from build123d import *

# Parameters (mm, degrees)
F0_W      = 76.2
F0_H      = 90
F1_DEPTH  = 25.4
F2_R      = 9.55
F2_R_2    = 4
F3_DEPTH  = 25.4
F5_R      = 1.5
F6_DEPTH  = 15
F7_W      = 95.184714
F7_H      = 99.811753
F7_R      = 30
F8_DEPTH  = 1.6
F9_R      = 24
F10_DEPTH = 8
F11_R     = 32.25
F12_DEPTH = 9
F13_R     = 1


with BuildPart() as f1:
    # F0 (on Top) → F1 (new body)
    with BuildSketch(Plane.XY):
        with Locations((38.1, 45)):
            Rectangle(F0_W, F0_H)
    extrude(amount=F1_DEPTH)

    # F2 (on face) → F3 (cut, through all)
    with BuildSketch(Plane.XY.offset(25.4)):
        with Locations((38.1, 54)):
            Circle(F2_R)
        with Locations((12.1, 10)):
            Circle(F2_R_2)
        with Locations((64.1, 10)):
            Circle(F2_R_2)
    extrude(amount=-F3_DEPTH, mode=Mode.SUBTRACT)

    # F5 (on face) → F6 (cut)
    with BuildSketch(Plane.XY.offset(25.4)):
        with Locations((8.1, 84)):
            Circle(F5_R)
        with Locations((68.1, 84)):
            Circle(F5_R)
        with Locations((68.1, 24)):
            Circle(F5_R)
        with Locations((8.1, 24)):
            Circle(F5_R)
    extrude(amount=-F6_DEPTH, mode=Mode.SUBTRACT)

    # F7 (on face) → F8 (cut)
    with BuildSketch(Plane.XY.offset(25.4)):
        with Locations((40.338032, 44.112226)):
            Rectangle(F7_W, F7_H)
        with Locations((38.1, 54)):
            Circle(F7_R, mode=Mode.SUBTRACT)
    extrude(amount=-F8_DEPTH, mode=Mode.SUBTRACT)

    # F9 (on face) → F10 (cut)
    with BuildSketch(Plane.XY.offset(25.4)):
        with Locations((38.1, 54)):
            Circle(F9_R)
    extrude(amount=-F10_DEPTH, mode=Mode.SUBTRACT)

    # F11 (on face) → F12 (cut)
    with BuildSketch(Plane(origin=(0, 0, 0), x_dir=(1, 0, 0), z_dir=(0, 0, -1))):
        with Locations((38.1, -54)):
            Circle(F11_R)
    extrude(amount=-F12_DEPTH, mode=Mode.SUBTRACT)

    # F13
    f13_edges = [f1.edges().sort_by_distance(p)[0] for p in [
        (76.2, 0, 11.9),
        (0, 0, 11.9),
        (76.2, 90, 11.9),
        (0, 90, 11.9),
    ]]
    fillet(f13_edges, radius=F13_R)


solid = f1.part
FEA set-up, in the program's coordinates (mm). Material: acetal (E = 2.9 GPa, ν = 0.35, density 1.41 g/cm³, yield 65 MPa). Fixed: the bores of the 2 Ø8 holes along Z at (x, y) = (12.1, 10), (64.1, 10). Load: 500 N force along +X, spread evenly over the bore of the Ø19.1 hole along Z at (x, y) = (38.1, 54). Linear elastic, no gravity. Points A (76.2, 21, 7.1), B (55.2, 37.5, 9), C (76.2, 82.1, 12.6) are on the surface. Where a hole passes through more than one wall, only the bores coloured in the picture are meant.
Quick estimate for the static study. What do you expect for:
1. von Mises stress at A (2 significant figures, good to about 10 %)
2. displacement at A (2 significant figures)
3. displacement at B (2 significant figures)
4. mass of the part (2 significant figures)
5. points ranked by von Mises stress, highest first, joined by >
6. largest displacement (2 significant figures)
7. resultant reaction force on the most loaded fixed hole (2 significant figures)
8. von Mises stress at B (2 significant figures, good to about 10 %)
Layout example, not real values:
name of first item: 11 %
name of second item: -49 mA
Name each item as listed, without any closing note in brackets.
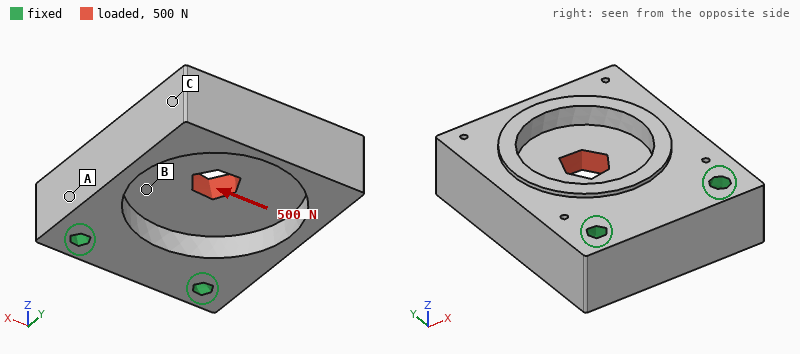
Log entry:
von Mises stress at A: 0.87 MPa
displacement at A: 9.3 µm
displacement at B: 18 µm
mass of the part: 170 g
points ranked by von Mises stress, highest first, joined by >: B > A > C
largest displacement: 59 µm
resultant reaction force on the most loaded fixed hole: 450 N
von Mises stress at B: 1.3 MPa
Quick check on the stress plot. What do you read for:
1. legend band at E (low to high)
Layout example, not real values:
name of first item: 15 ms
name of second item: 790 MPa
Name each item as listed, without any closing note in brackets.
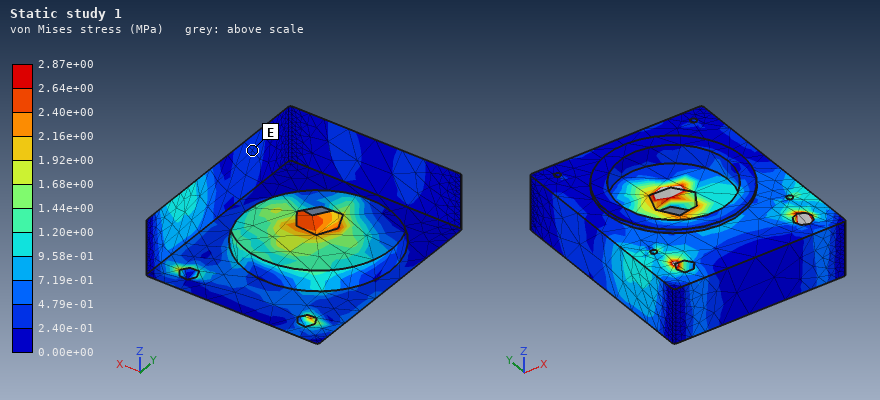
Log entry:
legend band at E: 2.40e-01 to 4.79e-01 MPa
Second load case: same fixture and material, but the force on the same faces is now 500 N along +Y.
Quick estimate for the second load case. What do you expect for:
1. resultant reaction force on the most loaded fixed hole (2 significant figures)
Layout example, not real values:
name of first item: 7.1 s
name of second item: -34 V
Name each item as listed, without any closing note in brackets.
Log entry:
resultant reaction force on the most loaded fixed hole: 260 N
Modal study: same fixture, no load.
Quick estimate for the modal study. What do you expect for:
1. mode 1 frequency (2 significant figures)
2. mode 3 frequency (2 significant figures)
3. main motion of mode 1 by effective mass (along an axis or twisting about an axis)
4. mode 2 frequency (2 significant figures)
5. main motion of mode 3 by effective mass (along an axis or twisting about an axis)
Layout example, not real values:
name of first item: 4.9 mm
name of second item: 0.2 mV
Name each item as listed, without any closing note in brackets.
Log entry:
mode 1 frequency: 650 Hz
mode 3 frequency: 1500 Hz
main motion of mode 1 by effective mass: along Z
mode 2 frequency: 1200 Hz
main motion of mode 3 by effective mass: along X
